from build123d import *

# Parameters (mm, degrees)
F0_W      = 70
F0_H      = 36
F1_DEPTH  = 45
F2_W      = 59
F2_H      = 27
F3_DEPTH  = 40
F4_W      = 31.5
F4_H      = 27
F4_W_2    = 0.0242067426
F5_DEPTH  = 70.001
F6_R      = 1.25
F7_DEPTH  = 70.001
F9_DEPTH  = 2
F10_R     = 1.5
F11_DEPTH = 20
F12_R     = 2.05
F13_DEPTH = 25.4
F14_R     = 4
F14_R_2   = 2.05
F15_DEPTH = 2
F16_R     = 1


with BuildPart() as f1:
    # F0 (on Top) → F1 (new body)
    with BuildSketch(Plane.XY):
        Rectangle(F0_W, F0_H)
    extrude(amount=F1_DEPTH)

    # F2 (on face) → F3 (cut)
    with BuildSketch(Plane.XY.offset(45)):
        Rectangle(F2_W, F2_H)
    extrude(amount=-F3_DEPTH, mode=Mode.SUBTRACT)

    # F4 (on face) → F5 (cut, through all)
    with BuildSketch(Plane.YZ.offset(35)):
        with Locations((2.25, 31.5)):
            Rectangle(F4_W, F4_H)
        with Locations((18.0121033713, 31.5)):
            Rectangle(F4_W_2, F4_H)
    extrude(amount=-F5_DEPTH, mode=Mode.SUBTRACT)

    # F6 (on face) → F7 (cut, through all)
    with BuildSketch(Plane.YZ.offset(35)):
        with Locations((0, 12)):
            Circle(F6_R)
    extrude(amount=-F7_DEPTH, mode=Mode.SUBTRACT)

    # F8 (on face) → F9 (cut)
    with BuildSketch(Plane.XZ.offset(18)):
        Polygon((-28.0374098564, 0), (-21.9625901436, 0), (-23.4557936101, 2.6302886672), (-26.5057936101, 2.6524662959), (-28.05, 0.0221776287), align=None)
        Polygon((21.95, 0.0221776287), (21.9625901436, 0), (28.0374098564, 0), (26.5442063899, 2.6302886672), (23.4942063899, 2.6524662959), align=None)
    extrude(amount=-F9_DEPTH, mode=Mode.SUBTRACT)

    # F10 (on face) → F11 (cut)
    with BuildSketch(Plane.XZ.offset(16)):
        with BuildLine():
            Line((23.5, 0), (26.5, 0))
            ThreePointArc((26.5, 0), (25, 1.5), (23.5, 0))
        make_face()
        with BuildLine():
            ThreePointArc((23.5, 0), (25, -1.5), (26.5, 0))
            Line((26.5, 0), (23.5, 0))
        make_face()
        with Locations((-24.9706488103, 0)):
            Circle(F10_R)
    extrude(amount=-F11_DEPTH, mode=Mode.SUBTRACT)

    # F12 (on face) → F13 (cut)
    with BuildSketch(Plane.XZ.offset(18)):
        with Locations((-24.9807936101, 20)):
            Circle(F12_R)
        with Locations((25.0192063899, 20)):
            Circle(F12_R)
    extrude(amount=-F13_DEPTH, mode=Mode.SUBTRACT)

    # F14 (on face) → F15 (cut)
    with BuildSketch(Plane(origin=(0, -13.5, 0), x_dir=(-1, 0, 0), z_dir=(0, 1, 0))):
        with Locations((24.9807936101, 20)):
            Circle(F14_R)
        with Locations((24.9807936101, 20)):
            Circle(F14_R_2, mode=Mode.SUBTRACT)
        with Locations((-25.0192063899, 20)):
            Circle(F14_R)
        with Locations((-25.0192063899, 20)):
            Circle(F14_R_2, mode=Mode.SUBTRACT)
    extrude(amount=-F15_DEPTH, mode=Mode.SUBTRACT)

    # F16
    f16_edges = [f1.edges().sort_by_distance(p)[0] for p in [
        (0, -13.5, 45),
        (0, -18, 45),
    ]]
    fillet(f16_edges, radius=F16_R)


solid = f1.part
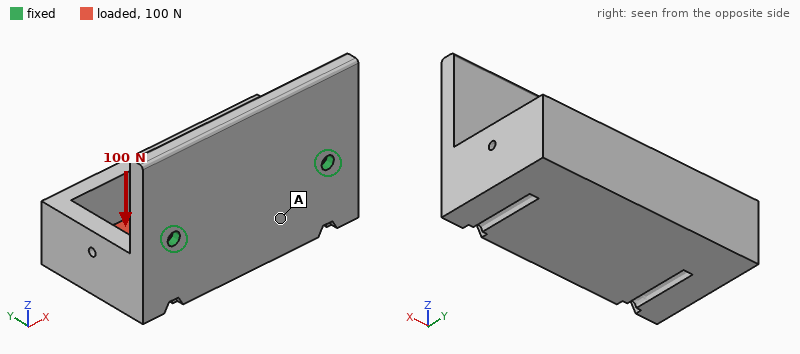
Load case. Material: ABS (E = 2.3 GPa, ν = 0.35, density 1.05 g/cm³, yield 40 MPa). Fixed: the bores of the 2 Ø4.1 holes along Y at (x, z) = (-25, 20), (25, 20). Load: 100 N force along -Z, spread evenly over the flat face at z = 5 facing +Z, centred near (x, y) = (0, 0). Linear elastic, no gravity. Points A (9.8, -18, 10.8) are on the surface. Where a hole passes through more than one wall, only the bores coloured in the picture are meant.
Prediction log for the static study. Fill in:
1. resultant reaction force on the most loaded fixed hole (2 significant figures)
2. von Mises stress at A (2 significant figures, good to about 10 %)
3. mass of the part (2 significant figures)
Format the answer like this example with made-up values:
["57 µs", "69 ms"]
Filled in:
["51 N", "2.7 MPa", "34 g"]
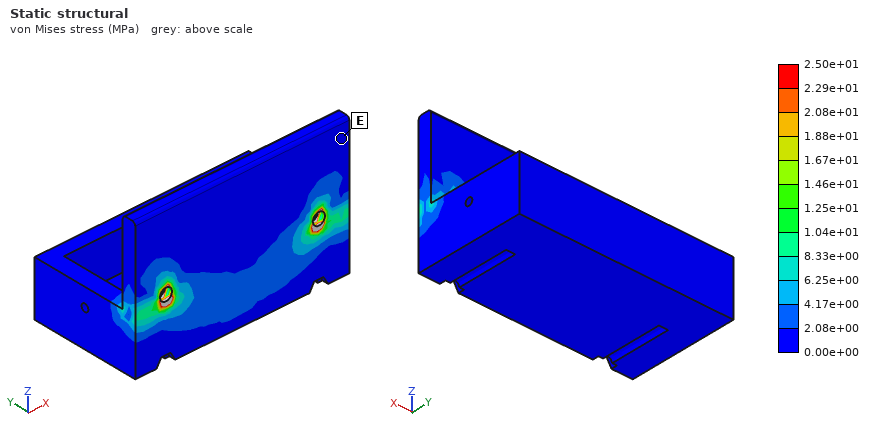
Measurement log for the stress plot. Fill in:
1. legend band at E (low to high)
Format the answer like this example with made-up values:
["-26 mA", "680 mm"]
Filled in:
["0.00e+00 to 2.08e+00 MPa"]
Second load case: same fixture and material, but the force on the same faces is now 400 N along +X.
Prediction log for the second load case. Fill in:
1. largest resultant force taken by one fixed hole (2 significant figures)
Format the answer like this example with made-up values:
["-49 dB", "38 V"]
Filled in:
["260 N"]
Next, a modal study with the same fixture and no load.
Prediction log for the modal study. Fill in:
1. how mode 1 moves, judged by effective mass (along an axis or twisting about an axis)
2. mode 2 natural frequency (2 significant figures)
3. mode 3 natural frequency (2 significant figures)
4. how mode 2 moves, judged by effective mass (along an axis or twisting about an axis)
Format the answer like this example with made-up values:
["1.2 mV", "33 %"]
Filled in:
["along Z", "700 Hz", "1200 Hz", "along X"]
